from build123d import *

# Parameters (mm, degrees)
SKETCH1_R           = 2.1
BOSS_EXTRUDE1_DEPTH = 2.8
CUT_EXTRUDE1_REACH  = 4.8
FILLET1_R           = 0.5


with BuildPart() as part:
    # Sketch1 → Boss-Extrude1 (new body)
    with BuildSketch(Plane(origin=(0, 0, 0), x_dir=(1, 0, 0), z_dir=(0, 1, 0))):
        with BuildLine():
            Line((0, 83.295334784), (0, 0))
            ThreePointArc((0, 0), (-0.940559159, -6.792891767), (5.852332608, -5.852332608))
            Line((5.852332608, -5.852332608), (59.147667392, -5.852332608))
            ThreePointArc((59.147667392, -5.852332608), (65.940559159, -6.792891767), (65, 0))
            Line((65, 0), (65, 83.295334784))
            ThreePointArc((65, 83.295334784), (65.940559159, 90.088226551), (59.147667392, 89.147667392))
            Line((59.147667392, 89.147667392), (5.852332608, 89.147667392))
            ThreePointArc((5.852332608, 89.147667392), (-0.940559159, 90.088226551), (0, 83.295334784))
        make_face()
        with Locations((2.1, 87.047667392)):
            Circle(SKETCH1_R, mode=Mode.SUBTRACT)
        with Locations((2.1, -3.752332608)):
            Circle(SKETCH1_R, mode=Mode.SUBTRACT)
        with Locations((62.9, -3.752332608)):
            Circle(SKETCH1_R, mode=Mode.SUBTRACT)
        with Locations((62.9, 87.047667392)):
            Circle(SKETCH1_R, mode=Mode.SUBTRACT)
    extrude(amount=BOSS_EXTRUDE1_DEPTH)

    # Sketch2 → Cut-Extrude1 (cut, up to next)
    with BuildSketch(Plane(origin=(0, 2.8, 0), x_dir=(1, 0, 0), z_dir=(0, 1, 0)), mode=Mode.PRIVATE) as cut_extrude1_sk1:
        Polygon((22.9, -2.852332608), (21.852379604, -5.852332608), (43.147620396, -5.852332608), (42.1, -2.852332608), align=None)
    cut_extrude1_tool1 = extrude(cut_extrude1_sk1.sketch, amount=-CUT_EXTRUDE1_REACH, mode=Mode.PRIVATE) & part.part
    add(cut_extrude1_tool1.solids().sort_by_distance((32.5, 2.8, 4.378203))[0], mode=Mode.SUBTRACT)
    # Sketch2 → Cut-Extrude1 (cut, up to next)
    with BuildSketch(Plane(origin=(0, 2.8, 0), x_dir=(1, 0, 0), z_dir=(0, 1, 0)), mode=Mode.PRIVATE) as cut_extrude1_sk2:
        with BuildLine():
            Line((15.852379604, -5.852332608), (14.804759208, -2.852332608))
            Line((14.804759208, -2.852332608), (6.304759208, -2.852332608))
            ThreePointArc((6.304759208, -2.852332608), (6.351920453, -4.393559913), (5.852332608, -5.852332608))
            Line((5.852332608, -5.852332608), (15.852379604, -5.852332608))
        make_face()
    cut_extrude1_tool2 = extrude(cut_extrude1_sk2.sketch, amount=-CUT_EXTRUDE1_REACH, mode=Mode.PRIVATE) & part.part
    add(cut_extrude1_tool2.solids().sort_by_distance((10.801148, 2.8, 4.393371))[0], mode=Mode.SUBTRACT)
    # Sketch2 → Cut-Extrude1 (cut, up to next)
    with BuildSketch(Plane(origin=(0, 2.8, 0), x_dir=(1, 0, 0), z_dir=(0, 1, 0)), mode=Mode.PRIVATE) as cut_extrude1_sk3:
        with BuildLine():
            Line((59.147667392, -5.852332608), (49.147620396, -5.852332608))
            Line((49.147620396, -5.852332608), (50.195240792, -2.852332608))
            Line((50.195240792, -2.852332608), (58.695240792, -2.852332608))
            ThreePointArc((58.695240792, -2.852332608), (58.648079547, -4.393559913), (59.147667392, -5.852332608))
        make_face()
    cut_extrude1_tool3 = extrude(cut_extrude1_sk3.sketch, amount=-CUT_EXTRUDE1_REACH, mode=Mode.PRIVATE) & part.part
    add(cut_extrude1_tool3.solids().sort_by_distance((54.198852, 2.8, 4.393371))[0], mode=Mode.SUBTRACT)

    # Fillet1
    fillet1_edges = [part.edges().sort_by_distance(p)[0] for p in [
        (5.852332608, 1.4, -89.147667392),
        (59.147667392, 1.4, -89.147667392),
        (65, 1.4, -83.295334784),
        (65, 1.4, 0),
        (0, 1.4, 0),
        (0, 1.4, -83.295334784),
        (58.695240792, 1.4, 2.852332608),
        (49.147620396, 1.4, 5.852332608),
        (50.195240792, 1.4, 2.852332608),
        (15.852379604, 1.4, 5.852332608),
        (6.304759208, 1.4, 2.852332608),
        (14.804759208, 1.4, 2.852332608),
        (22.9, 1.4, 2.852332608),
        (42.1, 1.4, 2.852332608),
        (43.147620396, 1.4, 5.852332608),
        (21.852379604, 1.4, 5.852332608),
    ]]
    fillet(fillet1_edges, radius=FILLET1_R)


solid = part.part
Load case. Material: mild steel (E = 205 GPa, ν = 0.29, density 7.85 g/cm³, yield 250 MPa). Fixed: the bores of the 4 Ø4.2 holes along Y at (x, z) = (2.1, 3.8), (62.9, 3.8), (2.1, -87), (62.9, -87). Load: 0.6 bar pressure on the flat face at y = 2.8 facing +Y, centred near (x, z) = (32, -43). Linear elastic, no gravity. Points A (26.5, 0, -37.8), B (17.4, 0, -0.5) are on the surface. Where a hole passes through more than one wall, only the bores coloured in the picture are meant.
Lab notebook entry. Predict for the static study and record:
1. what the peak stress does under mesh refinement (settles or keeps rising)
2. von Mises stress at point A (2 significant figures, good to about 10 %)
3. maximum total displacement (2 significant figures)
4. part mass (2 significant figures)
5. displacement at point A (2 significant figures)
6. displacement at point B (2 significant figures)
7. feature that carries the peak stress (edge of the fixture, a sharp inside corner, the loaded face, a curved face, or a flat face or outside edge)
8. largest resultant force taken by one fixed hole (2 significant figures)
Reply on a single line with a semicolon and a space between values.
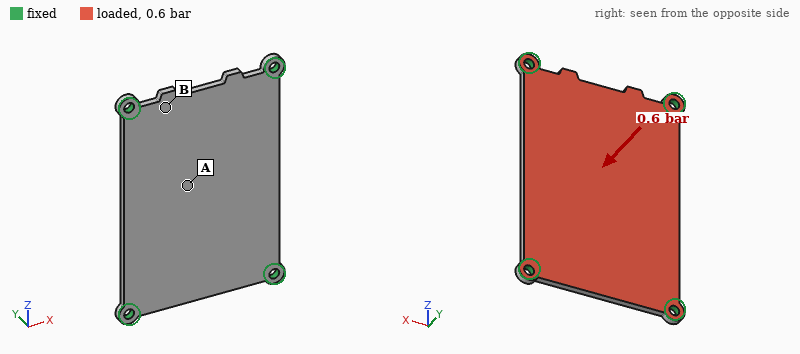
keeps rising; 18 MPa; 51 µm; 130 g; 51 µm; 9.6 µm; edge of the fixture; 94 N
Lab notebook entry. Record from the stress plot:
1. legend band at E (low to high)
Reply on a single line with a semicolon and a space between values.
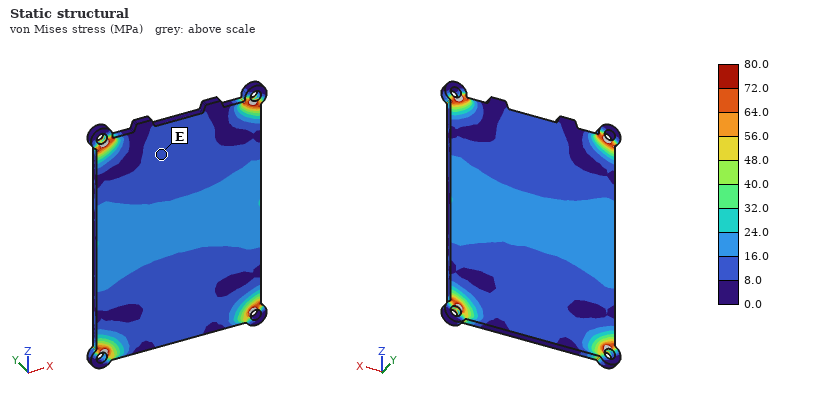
8.0 to 16.0 MPa
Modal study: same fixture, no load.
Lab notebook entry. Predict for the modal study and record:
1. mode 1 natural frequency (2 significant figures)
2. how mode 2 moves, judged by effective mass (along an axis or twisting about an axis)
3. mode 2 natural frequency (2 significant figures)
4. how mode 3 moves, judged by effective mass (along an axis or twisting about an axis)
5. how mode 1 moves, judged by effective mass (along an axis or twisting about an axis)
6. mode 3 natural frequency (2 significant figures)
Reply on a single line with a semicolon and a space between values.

1300 Hz; twisting about Z; 2400 Hz; twisting about X; along Y; 3300 Hz
